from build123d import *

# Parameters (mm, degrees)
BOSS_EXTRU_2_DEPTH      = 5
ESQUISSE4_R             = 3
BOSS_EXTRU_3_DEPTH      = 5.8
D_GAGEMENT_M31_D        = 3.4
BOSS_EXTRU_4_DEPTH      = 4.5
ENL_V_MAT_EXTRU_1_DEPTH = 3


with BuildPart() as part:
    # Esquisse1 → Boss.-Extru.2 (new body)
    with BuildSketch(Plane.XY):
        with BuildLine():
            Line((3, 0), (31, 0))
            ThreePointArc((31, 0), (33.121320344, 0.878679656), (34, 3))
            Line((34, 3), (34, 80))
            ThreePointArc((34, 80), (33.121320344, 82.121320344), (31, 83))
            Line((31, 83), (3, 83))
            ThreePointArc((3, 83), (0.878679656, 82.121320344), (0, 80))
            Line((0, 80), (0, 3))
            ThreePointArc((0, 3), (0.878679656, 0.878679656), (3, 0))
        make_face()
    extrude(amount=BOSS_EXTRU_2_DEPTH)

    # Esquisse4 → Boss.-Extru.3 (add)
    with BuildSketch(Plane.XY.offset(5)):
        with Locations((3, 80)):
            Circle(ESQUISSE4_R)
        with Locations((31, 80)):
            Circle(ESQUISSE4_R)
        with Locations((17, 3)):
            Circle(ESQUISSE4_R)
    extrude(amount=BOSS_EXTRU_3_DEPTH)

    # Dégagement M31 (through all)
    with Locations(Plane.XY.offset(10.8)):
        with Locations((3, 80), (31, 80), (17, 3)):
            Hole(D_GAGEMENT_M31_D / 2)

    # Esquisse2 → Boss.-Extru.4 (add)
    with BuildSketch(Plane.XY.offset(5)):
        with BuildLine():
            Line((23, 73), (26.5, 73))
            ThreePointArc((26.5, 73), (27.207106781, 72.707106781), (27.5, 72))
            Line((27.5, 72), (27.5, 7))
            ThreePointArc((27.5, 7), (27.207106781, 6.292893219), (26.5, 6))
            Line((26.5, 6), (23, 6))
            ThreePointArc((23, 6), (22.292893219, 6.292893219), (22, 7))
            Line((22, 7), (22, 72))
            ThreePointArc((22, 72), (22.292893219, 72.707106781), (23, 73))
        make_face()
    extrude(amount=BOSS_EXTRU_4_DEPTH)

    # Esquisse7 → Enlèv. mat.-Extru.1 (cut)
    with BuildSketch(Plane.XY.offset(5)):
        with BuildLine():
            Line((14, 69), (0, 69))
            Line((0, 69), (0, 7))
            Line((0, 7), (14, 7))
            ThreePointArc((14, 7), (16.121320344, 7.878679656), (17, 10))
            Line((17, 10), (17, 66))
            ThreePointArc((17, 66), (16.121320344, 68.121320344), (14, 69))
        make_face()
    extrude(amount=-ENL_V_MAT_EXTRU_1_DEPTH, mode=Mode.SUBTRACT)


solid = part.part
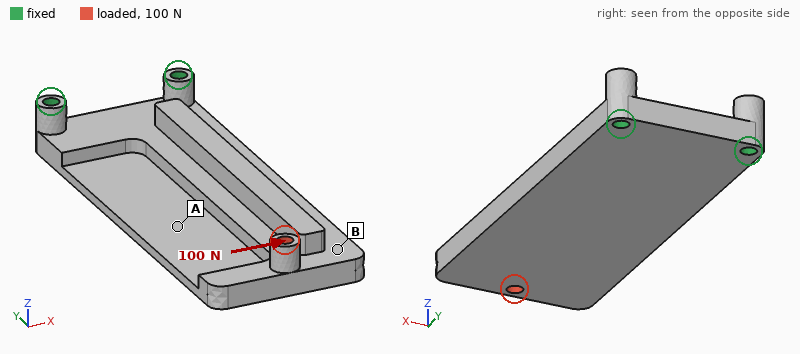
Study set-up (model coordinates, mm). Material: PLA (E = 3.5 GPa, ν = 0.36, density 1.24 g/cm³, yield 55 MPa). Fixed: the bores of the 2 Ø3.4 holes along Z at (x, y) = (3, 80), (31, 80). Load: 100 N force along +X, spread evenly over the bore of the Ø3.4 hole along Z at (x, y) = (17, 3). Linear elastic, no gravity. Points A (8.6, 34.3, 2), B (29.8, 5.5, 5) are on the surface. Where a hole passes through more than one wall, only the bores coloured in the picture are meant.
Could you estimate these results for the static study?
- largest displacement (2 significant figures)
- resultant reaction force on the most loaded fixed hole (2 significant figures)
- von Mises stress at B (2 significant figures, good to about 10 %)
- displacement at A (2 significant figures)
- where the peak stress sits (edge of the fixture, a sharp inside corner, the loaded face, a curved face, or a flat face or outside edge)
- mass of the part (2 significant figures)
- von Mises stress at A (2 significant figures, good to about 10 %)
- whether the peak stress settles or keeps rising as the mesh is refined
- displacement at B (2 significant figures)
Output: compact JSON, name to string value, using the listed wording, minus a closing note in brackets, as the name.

{"largest displacement": "1.00 mm", "resultant reaction force on the most loaded fixed hole": "280 N", "von Mises stress at B": "1.6 MPa", "displacement at A": "0.24 mm", "where the peak stress sits": "edge of the fixture", "mass of the part": "16 g", "von Mises stress at A": "5.5 MPa", "whether the peak stress settles or keeps rising as the mesh is refined": "keeps rising", "displacement at B": "0.87 mm"}
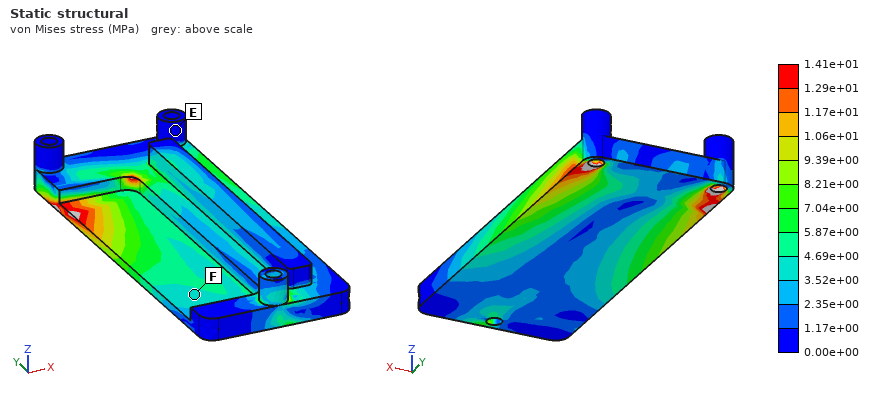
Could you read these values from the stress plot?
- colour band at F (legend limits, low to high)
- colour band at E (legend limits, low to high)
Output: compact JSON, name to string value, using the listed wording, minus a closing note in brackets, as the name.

{"colour band at F": "3.52e+00 to 4.69e+00 MPa", "colour band at E": "0.00e+00 to 1.17e+00 MPa"}
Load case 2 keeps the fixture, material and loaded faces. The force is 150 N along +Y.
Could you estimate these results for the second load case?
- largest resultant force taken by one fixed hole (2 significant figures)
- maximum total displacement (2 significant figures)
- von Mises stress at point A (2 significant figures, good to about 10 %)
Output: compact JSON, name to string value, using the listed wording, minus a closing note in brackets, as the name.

{"largest resultant force taken by one fixed hole": "81 N", "maximum total displacement": "1.0 mm", "von Mises stress at point A": "2.0 MPa"}
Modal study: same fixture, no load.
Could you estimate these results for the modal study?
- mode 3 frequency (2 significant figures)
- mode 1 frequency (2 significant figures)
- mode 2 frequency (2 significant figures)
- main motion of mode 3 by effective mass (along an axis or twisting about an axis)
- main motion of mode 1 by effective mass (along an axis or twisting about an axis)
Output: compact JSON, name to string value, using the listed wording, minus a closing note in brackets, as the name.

{"mode 3 frequency": "1100 Hz", "mode 1 frequency": "220 Hz", "mode 2 frequency": "920 Hz", "main motion of mode 3 by effective mass": "along X", "main motion of mode 1 by effective mass": "along Z"}
